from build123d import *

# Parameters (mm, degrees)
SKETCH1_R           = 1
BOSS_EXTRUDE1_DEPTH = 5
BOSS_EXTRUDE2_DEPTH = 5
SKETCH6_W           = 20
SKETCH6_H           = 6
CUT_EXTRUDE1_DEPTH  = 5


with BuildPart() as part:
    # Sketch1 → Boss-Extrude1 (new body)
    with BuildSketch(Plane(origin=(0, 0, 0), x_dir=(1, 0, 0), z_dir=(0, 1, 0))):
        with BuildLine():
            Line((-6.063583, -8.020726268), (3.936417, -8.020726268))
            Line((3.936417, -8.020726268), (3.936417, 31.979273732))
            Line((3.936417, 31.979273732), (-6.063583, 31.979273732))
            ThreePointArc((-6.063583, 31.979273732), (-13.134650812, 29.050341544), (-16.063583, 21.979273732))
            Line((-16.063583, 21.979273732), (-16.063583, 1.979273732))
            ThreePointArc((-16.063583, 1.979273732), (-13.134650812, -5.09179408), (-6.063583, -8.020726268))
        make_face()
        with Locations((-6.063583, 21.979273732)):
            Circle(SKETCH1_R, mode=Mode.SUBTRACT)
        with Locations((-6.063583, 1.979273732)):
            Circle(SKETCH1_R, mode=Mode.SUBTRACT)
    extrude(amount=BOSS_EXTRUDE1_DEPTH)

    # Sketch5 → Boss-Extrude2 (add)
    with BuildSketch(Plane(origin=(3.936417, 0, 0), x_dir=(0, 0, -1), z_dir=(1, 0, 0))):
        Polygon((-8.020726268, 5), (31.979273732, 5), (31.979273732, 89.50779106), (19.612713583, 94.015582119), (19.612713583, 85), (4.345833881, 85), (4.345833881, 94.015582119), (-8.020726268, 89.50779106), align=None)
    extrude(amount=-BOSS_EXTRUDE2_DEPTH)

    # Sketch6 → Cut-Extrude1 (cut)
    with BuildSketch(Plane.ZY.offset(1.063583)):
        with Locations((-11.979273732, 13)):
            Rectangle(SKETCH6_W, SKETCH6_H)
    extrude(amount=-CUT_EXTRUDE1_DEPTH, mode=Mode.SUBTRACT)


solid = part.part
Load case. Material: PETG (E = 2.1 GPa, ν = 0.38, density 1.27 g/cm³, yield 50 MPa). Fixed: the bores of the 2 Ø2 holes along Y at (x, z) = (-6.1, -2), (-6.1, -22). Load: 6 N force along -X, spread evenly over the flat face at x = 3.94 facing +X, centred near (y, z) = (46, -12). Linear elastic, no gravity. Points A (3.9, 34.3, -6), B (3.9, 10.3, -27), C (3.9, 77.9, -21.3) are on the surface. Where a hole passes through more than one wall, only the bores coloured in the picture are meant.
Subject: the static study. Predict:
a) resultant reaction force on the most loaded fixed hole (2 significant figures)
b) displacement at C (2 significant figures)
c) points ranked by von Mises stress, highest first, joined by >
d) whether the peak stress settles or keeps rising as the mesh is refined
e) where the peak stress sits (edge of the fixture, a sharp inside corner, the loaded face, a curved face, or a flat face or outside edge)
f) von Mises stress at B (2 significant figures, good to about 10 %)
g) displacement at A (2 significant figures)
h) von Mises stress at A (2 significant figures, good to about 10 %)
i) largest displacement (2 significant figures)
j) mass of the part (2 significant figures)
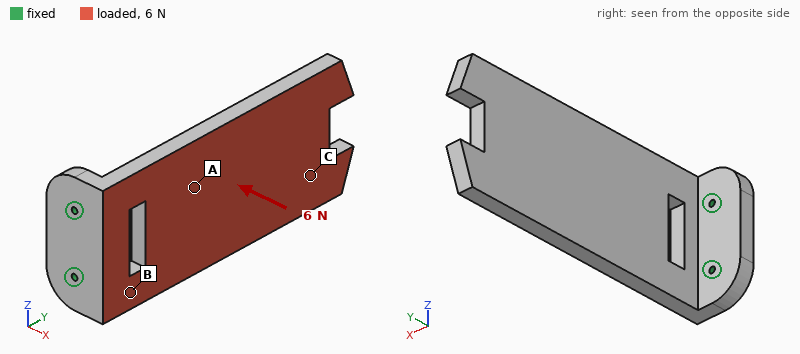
3.0 N
0.89 mm
B > A > C
keeps rising
edge of the fixture
2.3 MPa
0.28 mm
0.60 MPa
1.1 mm
25 g
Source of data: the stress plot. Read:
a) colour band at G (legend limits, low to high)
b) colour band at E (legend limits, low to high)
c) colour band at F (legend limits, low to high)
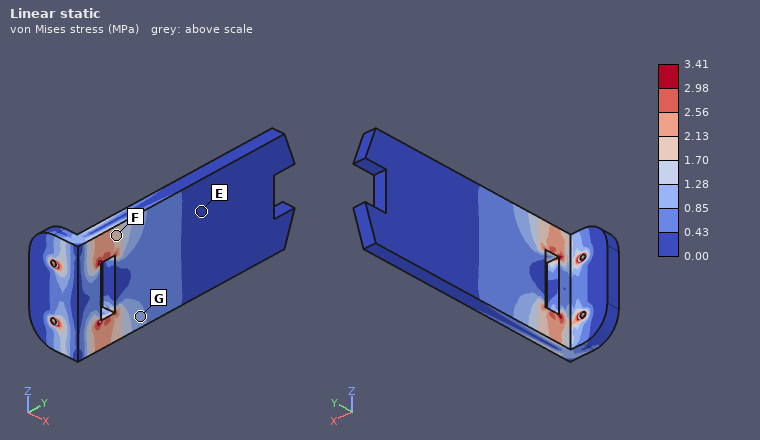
0.85 to 1.28 MPa
0.00 to 0.43 MPa
1.70 to 2.13 MPa
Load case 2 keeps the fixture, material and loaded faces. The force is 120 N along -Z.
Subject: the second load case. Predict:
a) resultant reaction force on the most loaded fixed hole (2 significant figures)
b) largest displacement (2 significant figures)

230 N
1.2 mm
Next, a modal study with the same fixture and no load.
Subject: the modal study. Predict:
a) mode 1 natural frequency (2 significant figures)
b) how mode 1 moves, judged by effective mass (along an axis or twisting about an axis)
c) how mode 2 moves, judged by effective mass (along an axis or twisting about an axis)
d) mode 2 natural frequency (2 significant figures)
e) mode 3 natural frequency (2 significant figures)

100 Hz
along X
along Z
400 Hz
560 Hz
